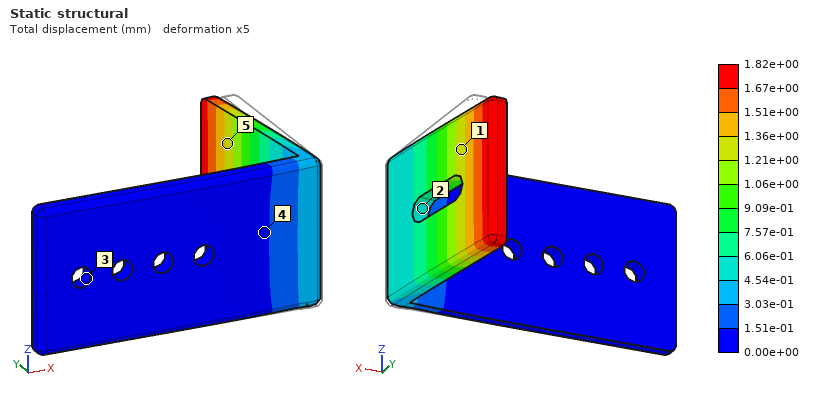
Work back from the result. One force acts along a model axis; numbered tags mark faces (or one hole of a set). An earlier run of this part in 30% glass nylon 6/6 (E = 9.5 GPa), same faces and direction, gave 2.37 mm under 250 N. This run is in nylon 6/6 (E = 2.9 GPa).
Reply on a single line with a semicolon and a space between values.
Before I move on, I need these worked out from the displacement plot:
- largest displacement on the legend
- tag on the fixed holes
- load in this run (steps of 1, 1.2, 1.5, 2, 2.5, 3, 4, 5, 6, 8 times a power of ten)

1.82e+00 mm; 3; 60 N
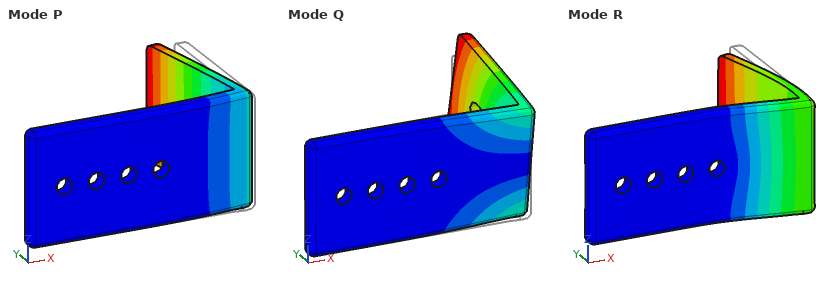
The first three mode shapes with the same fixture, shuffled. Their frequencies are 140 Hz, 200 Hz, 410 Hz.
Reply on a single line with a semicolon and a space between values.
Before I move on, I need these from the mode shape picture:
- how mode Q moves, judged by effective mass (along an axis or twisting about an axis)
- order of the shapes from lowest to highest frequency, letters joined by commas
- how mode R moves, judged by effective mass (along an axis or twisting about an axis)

along Z; P, Q, R; along Y
